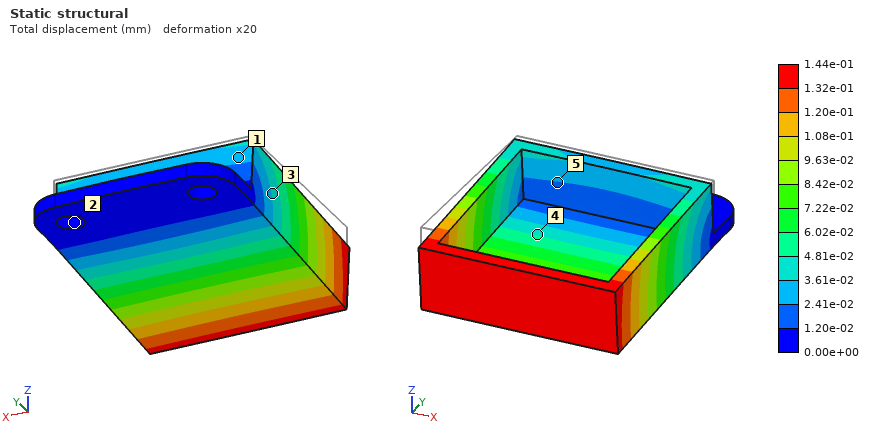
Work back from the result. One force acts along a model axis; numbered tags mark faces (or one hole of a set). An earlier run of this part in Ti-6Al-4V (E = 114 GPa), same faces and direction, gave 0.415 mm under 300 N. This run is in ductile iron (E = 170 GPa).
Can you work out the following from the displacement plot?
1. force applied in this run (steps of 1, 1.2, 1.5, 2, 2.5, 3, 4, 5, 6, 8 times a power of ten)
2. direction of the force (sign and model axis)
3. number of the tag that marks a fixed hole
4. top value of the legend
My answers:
150 N
-Z
2
1.44e-01 mm
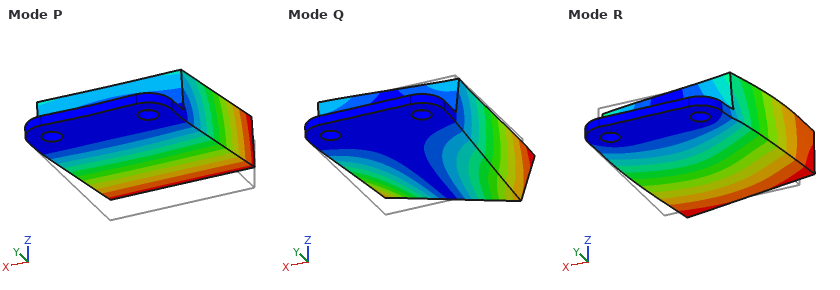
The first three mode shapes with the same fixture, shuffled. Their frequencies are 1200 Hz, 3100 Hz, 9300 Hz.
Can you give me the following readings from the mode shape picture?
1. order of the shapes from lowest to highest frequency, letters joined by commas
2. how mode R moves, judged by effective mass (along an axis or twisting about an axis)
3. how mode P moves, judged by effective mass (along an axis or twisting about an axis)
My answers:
P, Q, R
along X
along Z
